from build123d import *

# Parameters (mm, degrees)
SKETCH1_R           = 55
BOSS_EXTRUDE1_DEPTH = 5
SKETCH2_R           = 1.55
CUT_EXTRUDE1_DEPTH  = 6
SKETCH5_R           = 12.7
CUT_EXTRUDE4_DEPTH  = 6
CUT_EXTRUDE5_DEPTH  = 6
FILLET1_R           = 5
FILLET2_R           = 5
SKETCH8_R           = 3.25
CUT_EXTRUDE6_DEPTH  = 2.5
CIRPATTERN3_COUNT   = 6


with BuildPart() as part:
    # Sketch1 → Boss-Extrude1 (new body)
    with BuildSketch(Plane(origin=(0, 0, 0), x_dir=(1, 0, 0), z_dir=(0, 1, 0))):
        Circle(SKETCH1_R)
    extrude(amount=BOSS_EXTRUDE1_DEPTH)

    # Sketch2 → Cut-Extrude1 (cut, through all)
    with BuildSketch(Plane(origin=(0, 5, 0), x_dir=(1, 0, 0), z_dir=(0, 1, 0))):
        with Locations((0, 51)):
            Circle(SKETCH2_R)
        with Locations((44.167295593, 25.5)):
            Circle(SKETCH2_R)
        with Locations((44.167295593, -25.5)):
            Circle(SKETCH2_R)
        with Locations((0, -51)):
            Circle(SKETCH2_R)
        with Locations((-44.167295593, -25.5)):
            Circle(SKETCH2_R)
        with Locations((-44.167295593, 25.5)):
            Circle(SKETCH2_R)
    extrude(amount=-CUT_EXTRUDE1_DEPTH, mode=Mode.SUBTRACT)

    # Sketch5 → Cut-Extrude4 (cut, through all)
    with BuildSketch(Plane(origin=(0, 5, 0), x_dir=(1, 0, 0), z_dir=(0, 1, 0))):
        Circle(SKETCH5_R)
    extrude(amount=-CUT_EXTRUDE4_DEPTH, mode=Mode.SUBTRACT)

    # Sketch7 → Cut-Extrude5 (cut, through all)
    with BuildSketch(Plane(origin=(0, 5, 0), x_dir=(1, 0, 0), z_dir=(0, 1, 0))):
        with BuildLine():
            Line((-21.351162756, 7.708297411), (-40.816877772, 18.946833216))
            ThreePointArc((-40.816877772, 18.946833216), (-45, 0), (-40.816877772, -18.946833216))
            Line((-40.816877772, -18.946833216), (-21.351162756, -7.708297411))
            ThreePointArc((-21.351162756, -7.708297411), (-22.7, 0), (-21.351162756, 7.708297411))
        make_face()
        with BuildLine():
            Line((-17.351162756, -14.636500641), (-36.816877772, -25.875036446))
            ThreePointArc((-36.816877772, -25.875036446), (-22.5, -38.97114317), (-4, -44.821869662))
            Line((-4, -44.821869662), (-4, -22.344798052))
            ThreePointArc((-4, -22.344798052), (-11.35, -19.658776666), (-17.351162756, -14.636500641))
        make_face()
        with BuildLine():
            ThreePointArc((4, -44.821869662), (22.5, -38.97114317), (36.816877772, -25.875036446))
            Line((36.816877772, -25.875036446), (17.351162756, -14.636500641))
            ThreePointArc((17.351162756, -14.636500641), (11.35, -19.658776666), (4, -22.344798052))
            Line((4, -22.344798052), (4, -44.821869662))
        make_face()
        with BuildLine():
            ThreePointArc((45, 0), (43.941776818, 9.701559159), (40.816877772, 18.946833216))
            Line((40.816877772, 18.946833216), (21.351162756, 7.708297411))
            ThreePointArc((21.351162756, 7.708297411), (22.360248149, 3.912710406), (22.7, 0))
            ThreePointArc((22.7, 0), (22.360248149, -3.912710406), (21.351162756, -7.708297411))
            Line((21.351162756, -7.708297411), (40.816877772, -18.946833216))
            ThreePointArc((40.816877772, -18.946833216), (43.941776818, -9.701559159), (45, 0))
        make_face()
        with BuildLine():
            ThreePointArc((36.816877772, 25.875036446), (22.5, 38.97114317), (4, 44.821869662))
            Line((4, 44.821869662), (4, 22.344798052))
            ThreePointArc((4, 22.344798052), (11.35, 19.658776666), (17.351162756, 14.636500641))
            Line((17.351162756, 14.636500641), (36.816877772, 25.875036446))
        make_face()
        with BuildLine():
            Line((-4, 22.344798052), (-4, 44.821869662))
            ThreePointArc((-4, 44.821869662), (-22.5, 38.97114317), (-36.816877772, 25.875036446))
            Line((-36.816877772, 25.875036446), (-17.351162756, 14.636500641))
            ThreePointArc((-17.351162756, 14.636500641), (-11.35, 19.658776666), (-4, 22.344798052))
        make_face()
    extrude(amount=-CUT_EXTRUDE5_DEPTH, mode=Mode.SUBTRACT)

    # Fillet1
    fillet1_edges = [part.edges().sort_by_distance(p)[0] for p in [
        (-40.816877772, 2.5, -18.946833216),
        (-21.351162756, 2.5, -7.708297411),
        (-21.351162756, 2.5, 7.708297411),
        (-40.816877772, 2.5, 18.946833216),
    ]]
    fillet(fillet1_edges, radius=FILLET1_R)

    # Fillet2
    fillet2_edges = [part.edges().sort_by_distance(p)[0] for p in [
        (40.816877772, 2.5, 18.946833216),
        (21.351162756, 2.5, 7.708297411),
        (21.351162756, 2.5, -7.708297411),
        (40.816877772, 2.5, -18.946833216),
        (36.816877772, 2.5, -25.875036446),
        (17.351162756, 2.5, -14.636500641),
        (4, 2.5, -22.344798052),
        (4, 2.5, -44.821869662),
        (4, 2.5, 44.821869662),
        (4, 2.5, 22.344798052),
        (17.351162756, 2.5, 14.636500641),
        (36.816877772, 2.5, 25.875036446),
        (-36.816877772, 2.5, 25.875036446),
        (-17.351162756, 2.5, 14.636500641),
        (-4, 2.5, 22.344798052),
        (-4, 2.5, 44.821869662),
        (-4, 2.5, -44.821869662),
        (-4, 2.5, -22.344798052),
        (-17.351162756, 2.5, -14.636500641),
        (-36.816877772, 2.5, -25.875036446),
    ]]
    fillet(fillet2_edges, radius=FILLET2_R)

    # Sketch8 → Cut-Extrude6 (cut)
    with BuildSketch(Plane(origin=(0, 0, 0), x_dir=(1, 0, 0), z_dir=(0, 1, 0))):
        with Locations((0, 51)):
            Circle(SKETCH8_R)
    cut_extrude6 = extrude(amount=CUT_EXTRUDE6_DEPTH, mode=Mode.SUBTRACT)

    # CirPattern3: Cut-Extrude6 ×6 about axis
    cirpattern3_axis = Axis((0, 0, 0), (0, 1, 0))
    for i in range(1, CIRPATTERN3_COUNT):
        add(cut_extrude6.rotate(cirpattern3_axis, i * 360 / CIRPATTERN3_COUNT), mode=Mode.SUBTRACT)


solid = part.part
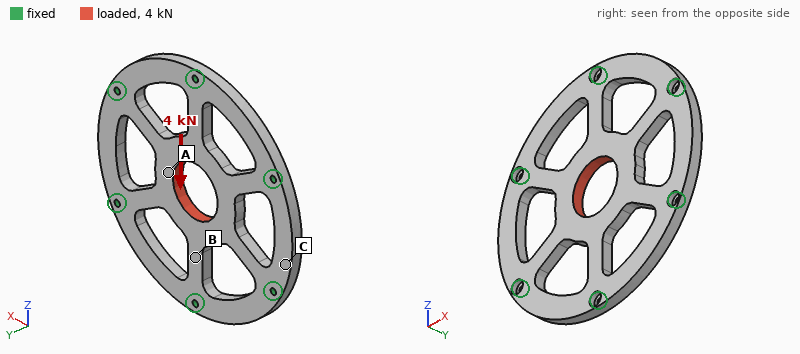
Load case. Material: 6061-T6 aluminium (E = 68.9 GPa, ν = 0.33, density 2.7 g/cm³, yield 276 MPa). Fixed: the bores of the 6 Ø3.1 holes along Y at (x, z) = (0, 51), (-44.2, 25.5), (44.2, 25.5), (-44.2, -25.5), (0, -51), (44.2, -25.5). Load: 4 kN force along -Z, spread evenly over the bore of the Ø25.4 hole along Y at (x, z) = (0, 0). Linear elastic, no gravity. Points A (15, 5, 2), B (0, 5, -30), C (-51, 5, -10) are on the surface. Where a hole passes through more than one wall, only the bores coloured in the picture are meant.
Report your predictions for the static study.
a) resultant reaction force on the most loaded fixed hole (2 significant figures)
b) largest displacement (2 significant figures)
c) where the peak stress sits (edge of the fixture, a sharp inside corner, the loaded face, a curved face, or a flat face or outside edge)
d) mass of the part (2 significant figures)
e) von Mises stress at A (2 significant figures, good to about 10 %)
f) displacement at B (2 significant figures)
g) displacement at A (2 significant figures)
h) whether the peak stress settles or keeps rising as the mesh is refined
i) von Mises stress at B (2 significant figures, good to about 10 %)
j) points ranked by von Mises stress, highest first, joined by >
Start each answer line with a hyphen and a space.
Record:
- 1.1 kN
- 19 µm
- edge of the fixture
- 72 g
- 19 MPa
- 14 µm
- 17 µm
- keeps rising
- 38 MPa
- B > A > C
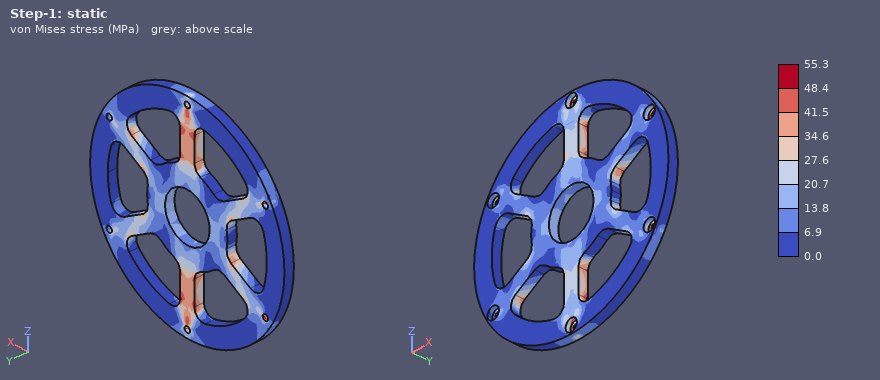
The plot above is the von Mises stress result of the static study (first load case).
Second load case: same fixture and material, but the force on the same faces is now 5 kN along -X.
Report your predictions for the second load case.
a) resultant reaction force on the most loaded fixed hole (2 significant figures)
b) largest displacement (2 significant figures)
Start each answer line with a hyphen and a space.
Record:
- 1.2 kN
- 25 µm
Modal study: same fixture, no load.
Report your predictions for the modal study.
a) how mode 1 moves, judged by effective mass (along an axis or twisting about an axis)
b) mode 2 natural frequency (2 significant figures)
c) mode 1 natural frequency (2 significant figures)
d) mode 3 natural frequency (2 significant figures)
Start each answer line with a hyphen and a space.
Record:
- along Y
- 5800 Hz
- 2800 Hz
- 5800 Hz
